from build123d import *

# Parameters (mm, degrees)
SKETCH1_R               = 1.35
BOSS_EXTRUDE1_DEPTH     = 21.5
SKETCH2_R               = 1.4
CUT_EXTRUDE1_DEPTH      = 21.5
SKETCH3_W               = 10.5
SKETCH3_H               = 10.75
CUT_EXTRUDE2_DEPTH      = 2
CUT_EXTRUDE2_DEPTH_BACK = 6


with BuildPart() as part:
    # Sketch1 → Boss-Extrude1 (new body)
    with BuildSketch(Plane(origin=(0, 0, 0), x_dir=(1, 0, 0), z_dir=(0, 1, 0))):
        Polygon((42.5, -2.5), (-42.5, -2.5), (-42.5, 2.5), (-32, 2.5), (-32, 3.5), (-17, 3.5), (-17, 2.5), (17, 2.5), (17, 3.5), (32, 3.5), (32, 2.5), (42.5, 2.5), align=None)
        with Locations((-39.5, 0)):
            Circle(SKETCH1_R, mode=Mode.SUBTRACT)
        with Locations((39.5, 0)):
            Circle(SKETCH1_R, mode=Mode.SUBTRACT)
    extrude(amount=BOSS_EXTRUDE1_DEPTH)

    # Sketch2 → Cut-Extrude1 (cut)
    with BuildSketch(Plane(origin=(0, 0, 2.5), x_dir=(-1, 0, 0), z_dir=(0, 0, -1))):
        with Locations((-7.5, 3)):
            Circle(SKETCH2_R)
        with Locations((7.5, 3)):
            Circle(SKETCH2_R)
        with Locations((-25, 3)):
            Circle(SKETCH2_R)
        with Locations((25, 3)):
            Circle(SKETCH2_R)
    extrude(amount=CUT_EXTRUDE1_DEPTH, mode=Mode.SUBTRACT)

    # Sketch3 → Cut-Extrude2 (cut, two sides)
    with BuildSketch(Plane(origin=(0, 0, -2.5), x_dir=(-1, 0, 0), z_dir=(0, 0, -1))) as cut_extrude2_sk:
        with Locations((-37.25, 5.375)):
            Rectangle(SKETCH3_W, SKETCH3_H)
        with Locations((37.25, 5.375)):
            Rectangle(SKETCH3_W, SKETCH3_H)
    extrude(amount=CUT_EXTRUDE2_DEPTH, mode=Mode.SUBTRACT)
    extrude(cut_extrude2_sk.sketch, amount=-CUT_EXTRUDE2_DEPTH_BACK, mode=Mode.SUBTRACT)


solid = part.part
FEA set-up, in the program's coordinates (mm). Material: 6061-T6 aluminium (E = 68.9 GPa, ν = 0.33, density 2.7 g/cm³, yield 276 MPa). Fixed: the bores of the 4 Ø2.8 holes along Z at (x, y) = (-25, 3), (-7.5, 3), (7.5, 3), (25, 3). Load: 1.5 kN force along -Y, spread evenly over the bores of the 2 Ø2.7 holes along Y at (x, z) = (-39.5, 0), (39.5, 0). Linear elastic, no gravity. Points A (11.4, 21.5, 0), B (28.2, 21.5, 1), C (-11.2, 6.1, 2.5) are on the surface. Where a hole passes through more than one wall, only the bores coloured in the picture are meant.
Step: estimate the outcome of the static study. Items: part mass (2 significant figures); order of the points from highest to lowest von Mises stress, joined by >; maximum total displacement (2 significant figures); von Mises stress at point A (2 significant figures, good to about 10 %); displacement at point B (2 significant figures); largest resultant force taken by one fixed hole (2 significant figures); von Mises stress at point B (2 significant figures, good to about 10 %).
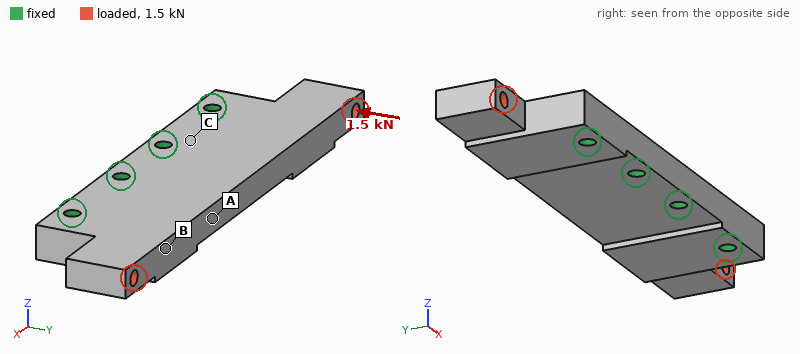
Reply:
23 g
B > A > C
34 µm
14 MPa
10 µm
1.1 kN
48 MPa
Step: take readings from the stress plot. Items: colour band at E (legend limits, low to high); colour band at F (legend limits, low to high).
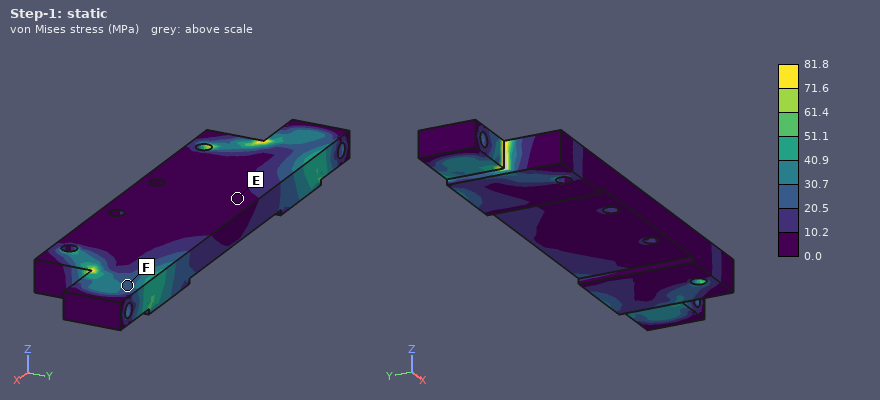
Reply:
0.0 to 10.2 MPa
20.5 to 30.7 MPa
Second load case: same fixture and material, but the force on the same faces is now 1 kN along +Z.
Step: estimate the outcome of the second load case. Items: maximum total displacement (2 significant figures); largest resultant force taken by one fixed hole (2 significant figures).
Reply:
0.13 mm
710 N
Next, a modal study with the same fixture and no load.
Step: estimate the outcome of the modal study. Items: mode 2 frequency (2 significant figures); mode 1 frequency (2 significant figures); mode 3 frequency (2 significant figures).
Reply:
9500 Hz
9300 Hz
12 kHz
